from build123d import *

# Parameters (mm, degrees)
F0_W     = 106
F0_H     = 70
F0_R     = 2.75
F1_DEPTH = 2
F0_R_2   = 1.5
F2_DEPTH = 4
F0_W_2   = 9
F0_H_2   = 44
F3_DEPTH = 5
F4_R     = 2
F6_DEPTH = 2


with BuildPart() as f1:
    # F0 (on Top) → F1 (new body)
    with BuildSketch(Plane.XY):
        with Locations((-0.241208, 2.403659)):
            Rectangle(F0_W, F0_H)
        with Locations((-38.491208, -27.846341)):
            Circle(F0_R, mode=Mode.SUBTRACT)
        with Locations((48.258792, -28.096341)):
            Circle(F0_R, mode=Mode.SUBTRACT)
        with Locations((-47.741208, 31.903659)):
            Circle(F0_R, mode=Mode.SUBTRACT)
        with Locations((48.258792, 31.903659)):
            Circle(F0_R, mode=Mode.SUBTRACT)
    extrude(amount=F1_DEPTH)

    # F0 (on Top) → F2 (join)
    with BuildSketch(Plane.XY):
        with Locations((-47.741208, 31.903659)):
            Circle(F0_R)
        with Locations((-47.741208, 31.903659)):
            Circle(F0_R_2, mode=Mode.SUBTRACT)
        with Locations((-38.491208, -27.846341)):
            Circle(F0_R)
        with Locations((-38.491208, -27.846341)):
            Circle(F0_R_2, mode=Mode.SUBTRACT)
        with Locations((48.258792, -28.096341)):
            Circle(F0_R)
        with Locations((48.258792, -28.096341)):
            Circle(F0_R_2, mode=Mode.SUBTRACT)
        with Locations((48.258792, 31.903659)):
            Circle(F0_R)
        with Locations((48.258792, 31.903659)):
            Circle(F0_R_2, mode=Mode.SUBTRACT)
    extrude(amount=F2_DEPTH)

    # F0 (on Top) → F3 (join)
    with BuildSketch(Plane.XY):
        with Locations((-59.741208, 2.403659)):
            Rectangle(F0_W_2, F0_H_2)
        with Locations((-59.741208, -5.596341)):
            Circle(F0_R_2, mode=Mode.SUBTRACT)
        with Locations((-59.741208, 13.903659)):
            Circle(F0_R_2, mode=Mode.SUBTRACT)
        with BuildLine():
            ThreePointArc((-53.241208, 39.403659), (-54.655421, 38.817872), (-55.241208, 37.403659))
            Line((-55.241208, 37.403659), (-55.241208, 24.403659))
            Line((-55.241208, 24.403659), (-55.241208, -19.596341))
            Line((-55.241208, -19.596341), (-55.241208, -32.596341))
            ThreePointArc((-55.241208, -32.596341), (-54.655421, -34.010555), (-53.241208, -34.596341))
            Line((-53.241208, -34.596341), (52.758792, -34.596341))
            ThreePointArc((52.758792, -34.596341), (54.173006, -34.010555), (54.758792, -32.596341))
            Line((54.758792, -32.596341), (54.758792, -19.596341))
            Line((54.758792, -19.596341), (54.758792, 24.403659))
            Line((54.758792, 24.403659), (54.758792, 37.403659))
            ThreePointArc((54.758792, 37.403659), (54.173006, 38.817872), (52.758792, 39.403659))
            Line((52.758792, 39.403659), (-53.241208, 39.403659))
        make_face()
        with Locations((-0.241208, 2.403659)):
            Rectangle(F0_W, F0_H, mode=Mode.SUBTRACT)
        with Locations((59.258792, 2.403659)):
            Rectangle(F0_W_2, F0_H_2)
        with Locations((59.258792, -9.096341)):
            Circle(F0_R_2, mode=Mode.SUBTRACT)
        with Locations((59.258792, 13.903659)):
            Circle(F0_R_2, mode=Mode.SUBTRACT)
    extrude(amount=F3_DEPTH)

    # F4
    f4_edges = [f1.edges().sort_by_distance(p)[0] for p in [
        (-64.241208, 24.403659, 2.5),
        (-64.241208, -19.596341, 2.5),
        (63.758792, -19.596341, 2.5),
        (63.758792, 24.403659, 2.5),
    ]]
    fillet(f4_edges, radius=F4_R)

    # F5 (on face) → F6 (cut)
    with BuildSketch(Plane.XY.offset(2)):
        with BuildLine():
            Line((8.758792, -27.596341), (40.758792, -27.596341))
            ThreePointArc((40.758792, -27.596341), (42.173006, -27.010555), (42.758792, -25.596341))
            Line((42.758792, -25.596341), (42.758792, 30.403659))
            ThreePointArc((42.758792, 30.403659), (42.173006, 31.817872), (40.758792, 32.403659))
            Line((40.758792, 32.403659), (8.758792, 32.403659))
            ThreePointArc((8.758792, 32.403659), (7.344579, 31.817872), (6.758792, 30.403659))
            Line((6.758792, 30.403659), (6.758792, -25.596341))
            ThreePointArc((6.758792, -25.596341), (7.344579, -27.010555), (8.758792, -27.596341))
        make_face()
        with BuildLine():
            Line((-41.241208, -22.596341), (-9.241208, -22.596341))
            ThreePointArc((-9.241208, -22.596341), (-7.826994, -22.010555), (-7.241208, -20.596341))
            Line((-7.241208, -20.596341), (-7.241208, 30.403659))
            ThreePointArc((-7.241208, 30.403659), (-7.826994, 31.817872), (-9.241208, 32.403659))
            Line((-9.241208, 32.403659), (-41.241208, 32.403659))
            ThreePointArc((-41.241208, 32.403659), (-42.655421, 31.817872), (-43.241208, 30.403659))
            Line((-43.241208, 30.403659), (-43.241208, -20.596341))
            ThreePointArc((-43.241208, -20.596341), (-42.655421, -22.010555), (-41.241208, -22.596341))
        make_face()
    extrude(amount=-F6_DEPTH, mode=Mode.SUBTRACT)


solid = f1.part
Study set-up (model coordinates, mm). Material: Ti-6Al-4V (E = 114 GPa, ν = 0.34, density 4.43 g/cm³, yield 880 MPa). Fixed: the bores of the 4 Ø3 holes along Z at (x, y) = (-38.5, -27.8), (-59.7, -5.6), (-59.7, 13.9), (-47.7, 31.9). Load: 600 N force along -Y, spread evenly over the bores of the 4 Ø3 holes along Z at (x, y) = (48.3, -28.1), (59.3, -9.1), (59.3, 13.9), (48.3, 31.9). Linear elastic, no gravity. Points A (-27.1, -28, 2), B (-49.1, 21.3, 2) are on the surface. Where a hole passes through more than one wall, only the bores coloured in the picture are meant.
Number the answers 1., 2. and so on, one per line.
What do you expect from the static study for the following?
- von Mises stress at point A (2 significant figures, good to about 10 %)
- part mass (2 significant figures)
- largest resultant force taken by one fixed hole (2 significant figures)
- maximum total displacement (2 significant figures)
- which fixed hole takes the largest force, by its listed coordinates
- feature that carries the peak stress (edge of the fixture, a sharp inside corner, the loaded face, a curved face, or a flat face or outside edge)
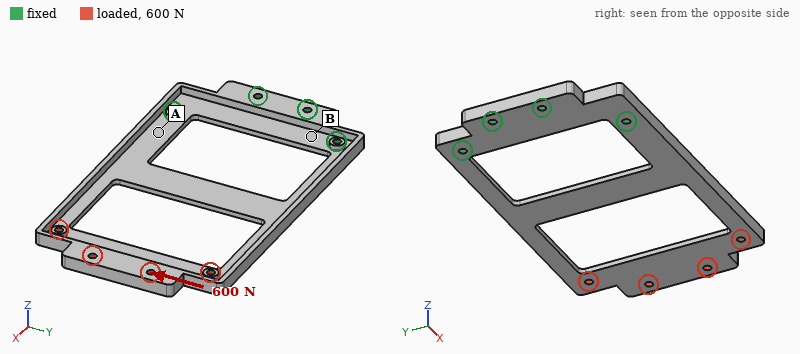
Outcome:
1. 71 MPa
2. 62 g
3. 1.1 kN
4. 0.92 mm
5. (-38.5, -27.8)
6. a curved face
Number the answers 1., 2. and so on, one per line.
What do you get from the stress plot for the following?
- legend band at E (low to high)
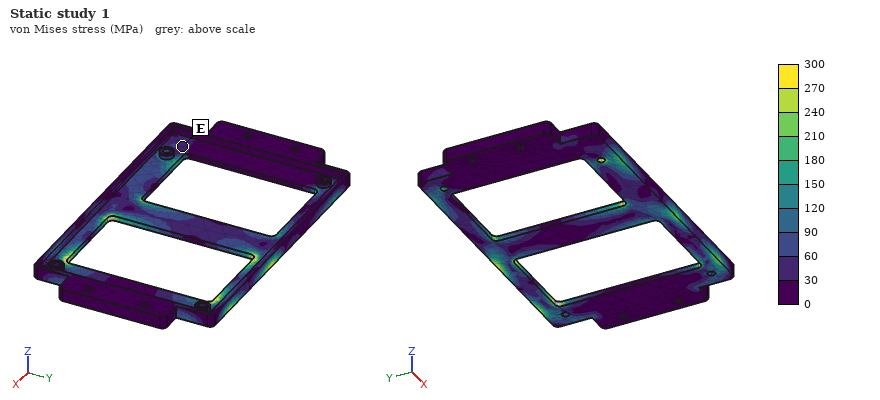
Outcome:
1. 30 to 60 MPa
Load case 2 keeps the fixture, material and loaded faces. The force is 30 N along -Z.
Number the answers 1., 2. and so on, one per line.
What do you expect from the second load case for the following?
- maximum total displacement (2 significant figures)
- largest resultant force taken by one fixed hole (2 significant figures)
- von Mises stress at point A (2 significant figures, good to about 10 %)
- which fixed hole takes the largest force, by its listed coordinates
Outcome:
1. 1.5 mm
2. 73 N
3. 24 MPa
4. (-38.5, -27.8)
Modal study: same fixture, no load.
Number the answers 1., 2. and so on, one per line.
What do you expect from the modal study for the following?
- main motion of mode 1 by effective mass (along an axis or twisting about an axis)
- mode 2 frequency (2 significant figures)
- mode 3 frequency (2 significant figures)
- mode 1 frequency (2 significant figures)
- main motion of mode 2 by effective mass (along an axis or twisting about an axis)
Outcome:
1. along Z
2. 470 Hz
3. 1000 Hz
4. 170 Hz
5. twisting about X
